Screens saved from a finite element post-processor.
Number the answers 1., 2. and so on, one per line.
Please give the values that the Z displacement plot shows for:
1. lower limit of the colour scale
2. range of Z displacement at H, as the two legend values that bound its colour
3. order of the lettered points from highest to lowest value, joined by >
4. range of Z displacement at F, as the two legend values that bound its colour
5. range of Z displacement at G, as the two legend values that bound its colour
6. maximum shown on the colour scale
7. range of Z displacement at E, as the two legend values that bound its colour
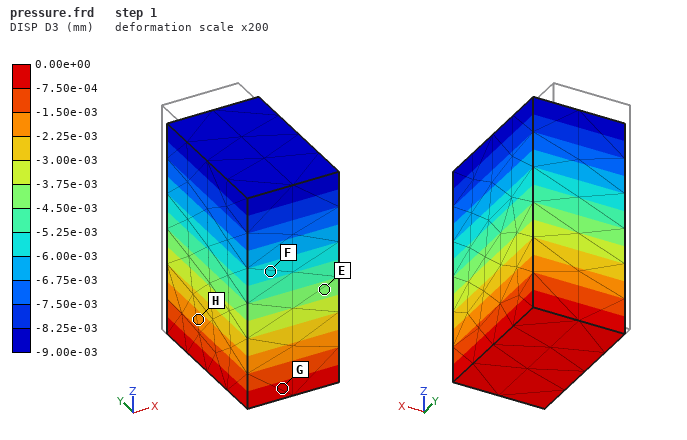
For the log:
1. -9.00e-03 mm
2. -2.25e-03 to -1.50e-03 mm
3. G > H > E > F
4. -6.00e-03 to -5.25e-03 mm
5. -7.50e-04 to 0.00e+00 mm
6. 0.00e+00 mm
7. -4.50e-03 to -3.75e-03 mm
